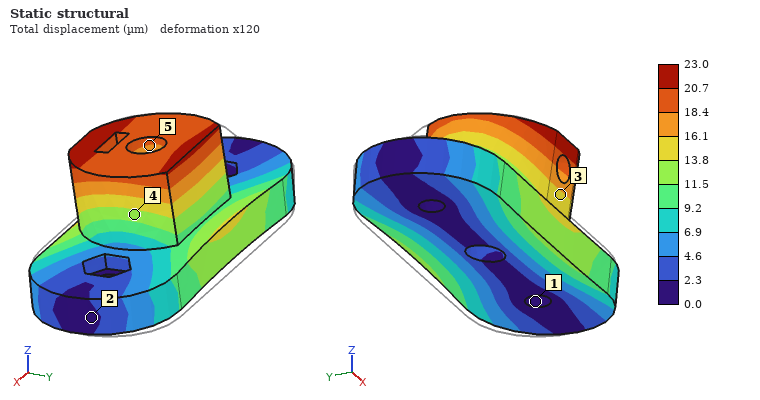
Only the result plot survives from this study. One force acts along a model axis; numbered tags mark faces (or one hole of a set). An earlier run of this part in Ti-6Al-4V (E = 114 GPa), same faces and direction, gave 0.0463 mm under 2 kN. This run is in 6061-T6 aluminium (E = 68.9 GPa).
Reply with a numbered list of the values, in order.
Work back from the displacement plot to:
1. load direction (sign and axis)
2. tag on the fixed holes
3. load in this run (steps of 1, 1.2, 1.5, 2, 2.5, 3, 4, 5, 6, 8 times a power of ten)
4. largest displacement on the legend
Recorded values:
1. -Y
2. 1
3. 600 N
4. 23.0 µm
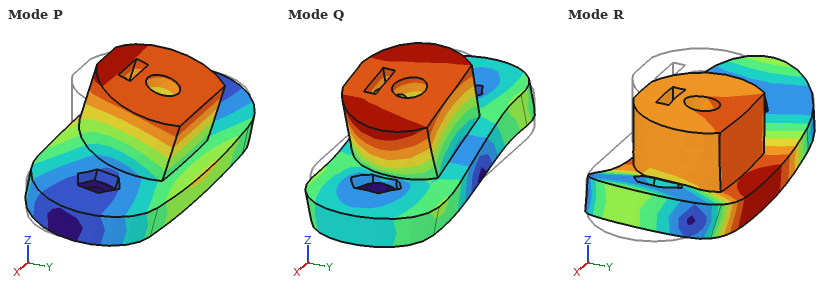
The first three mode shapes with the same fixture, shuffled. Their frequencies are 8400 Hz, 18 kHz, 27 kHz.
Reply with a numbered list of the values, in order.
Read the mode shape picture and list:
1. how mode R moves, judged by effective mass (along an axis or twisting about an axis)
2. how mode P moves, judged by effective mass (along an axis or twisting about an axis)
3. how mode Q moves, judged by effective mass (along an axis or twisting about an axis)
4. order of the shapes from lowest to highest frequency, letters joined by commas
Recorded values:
1. along Z
2. along Y
3. along X
4. P, R, Q
